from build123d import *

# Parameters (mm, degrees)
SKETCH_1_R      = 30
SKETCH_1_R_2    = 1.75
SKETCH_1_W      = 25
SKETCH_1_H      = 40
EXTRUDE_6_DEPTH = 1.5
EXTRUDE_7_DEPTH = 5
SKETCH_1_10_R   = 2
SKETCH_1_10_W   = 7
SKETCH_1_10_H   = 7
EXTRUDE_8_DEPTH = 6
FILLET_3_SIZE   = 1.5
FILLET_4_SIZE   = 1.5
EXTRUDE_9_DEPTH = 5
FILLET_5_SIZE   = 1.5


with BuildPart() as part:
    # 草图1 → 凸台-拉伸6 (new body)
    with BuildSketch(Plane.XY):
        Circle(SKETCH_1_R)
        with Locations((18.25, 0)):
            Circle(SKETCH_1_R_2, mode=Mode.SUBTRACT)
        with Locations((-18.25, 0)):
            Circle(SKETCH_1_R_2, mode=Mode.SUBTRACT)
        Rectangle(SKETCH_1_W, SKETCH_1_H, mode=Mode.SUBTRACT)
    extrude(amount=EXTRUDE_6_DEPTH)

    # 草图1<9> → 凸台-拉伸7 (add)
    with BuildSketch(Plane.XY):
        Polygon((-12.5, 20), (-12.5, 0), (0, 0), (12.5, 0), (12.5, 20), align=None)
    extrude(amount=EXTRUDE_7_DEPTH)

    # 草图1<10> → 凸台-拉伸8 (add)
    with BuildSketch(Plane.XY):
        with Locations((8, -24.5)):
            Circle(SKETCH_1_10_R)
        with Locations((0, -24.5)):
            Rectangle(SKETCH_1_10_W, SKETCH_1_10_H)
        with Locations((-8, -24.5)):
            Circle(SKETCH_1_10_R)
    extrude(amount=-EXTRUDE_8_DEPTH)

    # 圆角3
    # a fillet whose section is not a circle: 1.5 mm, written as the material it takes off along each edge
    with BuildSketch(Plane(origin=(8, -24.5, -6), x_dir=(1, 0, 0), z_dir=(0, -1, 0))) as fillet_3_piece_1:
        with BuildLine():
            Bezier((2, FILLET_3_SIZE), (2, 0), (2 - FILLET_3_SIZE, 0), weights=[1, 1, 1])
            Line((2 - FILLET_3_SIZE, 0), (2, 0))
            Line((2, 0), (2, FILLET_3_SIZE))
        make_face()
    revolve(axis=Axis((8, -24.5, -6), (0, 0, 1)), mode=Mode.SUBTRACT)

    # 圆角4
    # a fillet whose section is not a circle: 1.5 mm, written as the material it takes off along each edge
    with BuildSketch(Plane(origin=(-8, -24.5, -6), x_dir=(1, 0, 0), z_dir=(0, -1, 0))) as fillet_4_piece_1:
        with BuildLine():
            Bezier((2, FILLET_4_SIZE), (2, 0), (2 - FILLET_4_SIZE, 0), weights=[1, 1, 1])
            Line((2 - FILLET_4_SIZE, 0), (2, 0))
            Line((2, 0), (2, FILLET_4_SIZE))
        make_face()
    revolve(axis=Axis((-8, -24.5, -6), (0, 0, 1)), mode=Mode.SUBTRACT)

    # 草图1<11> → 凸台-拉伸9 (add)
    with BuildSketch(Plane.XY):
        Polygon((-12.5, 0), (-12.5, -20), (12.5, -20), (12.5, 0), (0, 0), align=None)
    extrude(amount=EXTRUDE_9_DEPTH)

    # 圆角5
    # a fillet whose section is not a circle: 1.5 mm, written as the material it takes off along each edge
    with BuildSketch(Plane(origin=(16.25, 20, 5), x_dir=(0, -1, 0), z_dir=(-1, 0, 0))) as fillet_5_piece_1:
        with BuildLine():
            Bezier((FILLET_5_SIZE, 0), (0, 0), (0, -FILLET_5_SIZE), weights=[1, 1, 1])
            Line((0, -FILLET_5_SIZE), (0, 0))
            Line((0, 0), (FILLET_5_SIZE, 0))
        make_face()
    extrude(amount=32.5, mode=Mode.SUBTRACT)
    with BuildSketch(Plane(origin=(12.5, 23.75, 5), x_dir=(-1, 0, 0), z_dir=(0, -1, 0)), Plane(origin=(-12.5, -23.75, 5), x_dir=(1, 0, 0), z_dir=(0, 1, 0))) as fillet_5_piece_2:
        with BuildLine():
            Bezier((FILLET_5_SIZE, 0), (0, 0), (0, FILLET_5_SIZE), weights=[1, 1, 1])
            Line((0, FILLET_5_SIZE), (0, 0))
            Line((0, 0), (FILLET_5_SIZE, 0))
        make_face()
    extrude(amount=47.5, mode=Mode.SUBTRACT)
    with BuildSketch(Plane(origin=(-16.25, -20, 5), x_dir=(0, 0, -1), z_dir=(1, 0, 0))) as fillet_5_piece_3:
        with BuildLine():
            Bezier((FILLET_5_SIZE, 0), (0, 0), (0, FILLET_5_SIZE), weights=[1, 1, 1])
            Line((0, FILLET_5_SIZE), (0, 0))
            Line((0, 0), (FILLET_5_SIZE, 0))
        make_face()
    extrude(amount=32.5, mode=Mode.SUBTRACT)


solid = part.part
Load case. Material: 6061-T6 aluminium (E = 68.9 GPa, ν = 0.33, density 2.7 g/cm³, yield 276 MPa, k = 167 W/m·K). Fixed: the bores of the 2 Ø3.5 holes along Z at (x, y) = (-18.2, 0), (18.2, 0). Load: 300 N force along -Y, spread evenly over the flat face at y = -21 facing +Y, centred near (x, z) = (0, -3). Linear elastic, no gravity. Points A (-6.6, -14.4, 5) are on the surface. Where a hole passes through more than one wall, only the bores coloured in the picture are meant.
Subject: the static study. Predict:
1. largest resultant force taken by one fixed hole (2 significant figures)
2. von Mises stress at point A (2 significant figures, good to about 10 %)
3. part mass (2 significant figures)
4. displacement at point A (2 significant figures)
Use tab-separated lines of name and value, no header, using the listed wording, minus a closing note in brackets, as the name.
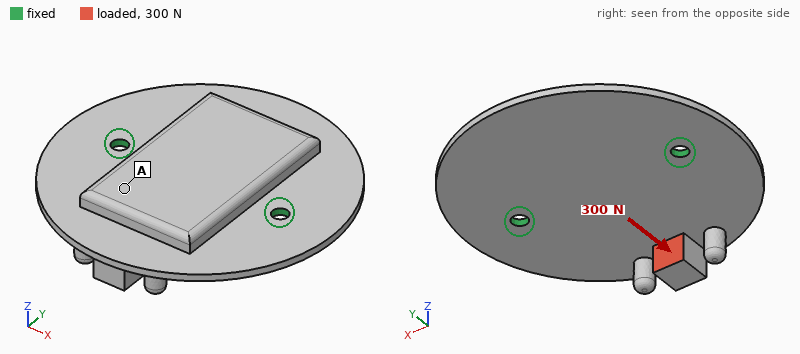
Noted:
largest resultant force taken by one fixed hole	160 N
von Mises stress at point A	13 MPa
part mass	22 g
displacement at point A	0.050 mm
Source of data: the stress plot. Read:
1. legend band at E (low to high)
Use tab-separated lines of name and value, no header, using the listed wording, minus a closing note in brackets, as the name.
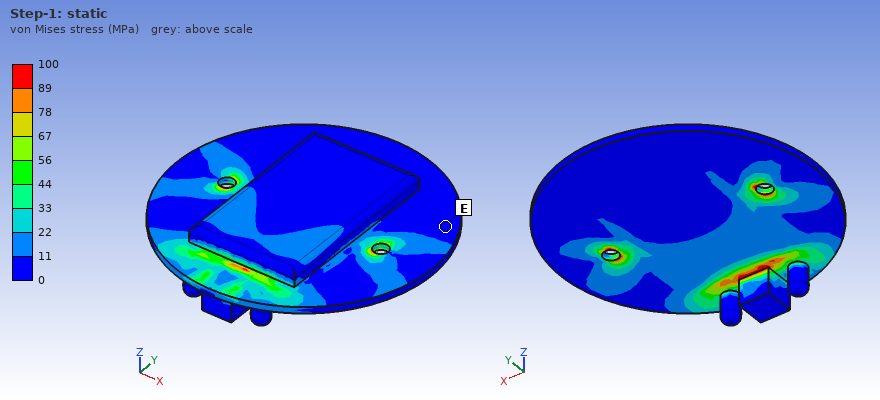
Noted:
legend band at E	0 to 11 MPa
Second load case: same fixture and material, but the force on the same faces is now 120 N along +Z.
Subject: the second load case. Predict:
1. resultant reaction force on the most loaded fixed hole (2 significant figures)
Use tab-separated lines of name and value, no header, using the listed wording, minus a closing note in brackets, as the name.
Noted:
resultant reaction force on the most loaded fixed hole	130 N
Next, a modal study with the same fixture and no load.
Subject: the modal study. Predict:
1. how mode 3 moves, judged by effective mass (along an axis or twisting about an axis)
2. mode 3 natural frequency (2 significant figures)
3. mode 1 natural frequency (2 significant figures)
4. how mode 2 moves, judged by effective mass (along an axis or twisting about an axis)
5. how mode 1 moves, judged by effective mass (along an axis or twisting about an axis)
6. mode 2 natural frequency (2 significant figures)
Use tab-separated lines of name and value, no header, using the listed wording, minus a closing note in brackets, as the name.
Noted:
how mode 3 moves, judged by effective mass	twisting about Y
mode 3 natural frequency	6900 Hz
mode 1 natural frequency	1500 Hz
how mode 2 moves, judged by effective mass	along Z
how mode 1 moves, judged by effective mass	twisting about X
mode 2 natural frequency	4200 Hz
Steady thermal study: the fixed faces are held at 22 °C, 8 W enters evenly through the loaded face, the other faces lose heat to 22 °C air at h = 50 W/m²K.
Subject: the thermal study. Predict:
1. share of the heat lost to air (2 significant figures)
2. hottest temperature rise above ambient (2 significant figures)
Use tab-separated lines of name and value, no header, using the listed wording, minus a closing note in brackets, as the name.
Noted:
share of the heat lost to air	21 %
hottest temperature rise above ambient	21 K
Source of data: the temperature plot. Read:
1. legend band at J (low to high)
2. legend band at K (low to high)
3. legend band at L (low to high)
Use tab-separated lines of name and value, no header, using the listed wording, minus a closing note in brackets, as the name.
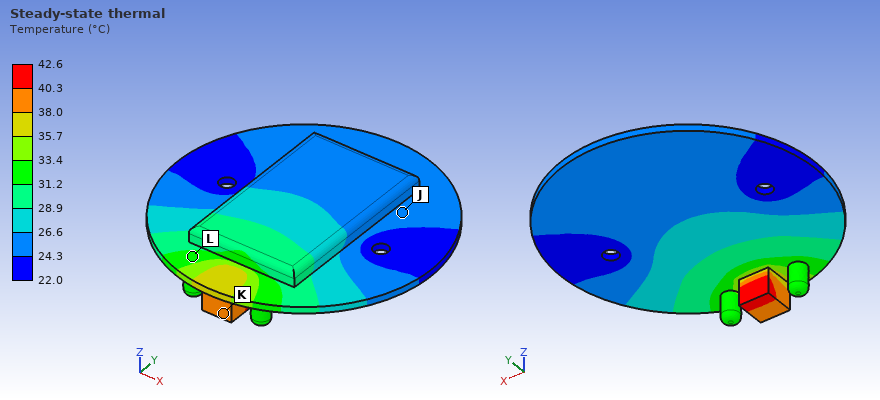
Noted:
legend band at J	24.3 to 26.6 °C
legend band at K	38.0 to 40.3 °C
legend band at L	31.2 to 33.4 °C
